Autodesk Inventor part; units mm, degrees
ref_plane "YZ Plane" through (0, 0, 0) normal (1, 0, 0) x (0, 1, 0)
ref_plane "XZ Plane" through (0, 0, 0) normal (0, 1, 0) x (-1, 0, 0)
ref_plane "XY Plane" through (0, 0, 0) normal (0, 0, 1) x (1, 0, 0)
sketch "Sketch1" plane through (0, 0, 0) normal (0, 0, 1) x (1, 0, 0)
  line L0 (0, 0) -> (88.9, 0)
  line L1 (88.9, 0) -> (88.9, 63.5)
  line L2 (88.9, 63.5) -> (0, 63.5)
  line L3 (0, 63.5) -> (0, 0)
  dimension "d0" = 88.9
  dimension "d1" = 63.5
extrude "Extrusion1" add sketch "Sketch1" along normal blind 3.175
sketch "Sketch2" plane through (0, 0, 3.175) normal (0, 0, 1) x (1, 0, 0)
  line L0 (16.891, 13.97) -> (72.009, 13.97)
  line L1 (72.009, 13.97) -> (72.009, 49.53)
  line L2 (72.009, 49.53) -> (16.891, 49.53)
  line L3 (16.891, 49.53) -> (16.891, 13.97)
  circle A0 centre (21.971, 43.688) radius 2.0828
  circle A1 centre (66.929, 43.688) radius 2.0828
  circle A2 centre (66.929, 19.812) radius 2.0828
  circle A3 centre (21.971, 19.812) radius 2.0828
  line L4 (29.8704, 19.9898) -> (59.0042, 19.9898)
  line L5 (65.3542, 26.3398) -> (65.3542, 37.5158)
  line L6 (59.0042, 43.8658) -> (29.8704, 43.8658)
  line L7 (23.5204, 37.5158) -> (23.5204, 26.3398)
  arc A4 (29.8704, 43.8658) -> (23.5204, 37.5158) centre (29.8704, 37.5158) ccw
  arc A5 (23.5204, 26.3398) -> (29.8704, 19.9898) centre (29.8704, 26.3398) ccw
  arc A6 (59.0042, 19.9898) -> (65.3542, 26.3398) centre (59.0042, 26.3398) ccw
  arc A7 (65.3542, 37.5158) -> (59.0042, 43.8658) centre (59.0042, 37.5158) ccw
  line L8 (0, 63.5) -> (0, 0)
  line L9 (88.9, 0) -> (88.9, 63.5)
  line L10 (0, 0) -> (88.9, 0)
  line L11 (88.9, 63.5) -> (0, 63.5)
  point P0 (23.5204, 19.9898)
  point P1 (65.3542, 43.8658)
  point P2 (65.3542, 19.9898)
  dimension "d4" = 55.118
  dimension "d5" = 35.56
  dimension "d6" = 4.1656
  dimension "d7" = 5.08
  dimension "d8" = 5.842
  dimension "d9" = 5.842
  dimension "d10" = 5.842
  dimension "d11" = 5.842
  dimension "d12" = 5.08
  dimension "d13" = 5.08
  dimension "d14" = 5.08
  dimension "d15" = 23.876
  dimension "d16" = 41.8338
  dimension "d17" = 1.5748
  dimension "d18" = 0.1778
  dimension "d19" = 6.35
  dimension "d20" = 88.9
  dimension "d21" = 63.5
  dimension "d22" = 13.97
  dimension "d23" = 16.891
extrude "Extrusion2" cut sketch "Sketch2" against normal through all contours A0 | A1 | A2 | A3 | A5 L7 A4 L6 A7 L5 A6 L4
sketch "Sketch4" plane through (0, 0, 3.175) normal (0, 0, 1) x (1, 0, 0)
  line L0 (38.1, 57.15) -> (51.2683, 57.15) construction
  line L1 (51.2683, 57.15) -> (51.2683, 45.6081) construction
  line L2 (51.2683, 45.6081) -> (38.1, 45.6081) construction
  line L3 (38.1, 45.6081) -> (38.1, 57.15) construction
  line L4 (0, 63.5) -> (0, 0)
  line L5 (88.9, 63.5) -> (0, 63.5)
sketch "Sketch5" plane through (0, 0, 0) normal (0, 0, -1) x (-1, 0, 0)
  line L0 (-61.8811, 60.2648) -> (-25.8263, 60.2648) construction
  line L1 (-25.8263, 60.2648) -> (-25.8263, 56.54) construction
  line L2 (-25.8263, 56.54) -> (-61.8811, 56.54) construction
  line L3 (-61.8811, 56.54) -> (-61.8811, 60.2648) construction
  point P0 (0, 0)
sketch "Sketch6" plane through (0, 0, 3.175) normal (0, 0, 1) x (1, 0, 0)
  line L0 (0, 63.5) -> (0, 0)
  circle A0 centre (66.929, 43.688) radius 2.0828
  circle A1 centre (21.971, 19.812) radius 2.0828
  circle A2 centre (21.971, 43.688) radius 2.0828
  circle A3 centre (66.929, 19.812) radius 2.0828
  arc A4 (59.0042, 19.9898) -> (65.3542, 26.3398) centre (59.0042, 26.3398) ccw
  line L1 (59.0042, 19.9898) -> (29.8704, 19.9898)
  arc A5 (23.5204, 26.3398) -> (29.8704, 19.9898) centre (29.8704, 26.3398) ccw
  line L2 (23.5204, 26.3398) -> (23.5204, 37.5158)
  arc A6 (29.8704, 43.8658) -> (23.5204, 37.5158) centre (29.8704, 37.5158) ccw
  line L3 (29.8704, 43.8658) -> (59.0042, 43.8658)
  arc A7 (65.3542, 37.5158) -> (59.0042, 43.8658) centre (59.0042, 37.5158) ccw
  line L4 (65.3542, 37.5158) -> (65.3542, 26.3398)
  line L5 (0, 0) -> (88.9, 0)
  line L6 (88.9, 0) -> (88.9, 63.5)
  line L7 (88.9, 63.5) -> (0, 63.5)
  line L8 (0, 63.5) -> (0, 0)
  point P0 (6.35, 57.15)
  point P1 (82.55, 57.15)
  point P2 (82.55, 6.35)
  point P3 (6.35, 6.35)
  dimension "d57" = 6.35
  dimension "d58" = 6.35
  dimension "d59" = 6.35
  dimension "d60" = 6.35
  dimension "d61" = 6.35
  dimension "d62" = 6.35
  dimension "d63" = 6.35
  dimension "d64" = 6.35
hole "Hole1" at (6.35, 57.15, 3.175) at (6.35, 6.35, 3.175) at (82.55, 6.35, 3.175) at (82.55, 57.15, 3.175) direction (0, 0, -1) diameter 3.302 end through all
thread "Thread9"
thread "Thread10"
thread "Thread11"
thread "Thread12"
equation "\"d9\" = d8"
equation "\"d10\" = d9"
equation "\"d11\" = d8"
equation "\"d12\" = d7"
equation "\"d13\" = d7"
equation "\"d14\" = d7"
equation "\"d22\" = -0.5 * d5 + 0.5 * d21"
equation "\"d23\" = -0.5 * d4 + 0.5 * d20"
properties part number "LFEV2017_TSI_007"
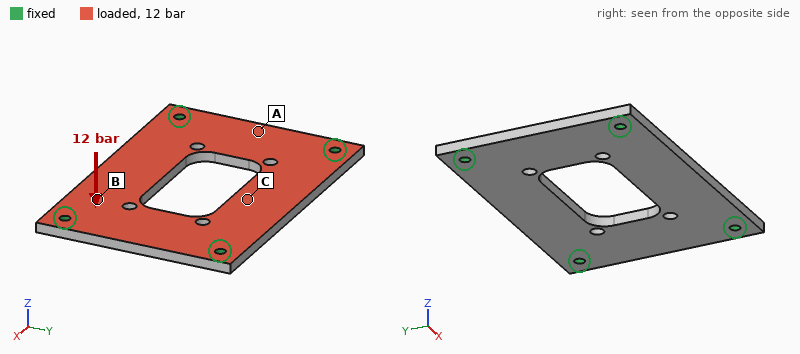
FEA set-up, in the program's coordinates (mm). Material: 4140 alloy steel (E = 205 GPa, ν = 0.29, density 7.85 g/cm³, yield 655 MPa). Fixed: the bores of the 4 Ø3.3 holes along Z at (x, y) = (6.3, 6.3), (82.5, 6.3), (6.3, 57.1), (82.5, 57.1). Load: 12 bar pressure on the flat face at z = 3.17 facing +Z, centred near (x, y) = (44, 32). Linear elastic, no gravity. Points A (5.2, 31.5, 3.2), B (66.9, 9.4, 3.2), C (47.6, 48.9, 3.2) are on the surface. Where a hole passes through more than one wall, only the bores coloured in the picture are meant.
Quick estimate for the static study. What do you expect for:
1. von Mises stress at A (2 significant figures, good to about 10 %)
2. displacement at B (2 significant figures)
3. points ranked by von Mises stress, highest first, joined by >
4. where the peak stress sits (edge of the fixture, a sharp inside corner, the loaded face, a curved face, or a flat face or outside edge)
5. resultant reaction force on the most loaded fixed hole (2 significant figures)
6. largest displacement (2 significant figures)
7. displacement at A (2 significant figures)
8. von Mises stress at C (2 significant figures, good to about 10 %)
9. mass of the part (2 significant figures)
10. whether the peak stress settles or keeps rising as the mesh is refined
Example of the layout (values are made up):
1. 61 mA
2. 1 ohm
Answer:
1. 92 MPa
2. 0.11 mm
3. C > A > B
4. edge of the fixture
5. 1.4 kN
6. 0.27 mm
7. 0.046 mm
8. 180 MPa
9. 110 g
10. keeps rising
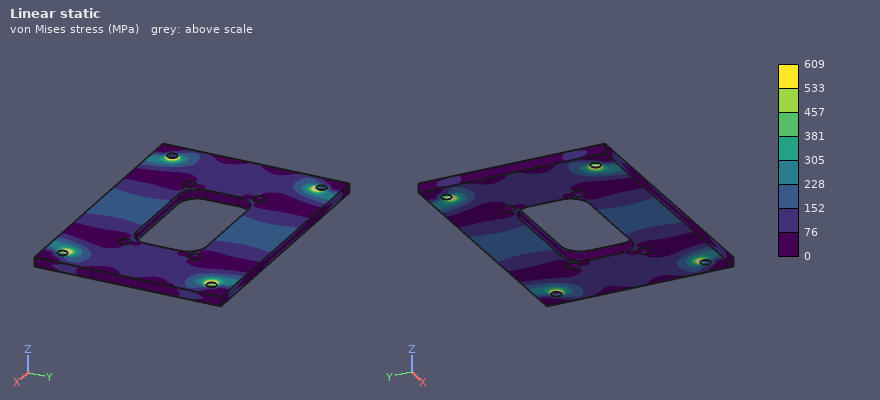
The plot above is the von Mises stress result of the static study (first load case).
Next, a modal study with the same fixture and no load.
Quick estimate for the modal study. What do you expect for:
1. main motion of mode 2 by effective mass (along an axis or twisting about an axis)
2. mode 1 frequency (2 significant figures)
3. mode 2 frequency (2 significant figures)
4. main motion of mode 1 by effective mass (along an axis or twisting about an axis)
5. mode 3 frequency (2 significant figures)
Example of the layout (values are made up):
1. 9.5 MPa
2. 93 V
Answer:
1. twisting about X
2. 2700 Hz
3. 3200 Hz
4. along Z
5. 5200 Hz
